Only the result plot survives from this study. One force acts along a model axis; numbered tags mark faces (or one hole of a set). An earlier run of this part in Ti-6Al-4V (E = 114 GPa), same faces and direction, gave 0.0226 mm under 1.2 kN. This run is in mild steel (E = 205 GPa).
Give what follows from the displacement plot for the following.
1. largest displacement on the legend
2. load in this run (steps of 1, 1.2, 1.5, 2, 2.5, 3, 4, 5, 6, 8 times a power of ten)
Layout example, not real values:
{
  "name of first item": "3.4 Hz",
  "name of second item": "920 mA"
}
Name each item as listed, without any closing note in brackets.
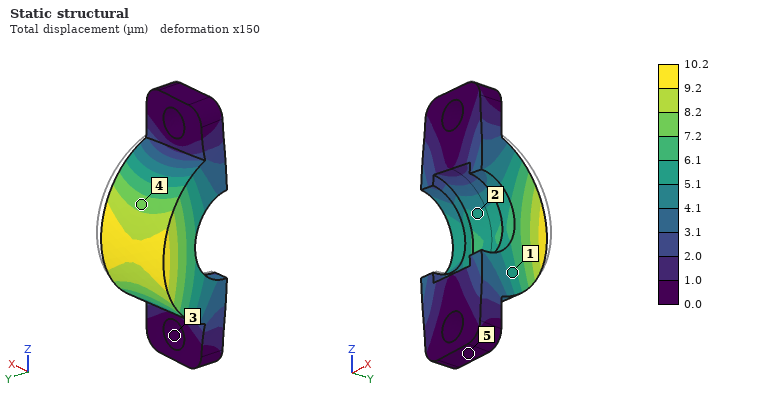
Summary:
{
  "largest displacement on the legend": "10.2 µm",
  "load in this run": "1 kN"
}
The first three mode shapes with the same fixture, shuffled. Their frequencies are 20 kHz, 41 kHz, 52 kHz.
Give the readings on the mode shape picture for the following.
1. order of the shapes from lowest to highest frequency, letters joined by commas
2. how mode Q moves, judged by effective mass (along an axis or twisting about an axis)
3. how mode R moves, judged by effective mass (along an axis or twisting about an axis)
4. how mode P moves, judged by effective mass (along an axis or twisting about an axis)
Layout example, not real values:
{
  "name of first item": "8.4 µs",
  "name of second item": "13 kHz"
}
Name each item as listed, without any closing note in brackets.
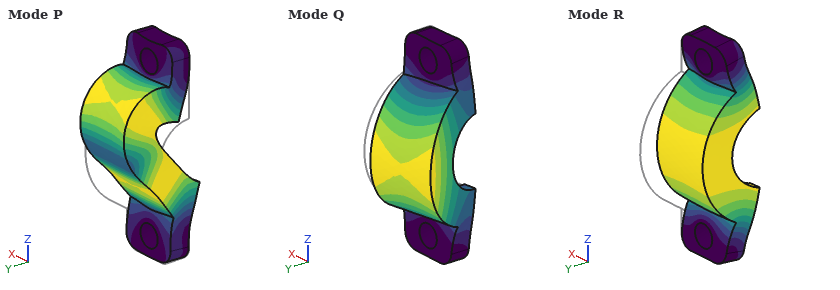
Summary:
{
  "order of the shapes from lowest to highest frequency, letters joined by commas": "Q, R, P",
  "how mode Q moves, judged by effective mass": "along X",
  "how mode R moves, judged by effective mass": "along Y",
  "how mode P moves, judged by effective mass": "along Z"
}
